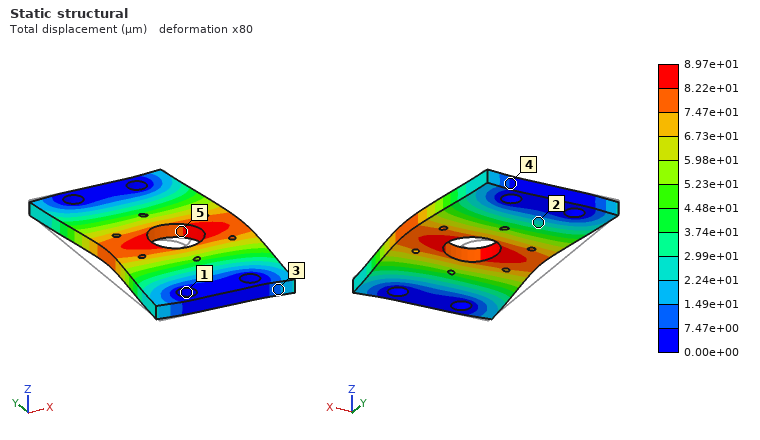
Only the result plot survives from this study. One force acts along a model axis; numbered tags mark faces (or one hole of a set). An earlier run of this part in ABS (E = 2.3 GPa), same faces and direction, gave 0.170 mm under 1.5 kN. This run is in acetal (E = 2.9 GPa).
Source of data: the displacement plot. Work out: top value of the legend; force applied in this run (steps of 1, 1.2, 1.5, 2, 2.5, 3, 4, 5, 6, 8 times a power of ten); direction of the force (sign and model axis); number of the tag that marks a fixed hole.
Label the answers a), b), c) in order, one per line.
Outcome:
a) 8.97e+01 µm
b) 1 kN
c) +X
d) 1
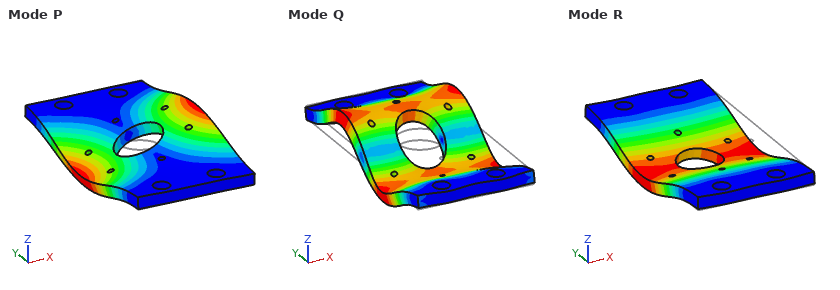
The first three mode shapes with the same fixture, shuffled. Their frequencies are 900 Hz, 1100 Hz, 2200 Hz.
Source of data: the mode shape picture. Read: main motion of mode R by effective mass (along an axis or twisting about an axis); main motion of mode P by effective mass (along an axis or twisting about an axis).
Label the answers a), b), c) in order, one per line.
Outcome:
a) along Z
b) twisting about Y
